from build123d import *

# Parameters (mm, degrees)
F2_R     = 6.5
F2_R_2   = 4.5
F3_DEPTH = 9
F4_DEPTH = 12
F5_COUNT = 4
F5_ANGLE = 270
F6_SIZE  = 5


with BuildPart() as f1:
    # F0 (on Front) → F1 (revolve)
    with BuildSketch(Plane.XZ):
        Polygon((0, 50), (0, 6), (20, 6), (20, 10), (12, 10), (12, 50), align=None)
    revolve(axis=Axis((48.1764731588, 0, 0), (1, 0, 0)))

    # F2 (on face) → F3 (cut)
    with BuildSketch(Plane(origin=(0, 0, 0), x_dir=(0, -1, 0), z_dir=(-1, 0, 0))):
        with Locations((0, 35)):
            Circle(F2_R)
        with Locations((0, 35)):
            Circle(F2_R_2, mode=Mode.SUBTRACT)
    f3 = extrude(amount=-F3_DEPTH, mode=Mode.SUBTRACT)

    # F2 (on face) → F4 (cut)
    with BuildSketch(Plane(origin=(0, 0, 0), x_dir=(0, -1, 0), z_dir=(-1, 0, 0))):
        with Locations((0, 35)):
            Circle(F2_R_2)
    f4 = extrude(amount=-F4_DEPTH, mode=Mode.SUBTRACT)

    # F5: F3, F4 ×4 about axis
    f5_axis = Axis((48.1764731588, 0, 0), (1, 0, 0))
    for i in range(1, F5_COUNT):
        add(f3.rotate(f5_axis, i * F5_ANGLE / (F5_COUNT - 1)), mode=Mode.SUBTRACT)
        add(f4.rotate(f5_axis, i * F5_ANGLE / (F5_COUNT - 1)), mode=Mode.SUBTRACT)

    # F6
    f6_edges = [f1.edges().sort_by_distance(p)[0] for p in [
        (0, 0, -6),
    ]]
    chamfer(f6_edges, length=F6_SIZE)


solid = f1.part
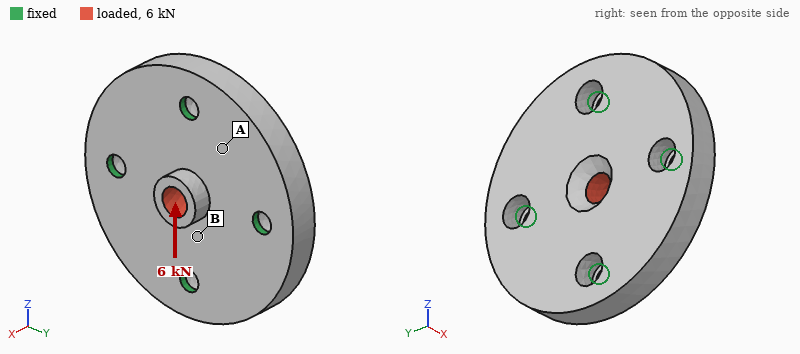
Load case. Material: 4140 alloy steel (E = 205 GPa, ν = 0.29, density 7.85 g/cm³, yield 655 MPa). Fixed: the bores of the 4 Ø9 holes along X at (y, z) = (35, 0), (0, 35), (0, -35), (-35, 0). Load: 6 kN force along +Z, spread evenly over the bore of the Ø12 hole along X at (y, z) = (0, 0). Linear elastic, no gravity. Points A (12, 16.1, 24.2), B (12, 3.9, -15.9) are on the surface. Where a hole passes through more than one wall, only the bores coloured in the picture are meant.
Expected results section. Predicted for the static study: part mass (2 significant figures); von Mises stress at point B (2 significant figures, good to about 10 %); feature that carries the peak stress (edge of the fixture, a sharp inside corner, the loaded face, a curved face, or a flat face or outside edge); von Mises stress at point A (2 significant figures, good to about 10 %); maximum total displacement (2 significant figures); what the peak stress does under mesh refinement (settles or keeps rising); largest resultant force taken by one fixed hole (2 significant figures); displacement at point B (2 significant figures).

690 g
19 MPa
edge of the fixture
5.5 MPa
5.9 µm
keeps rising
1.6 kN
1.7 µm
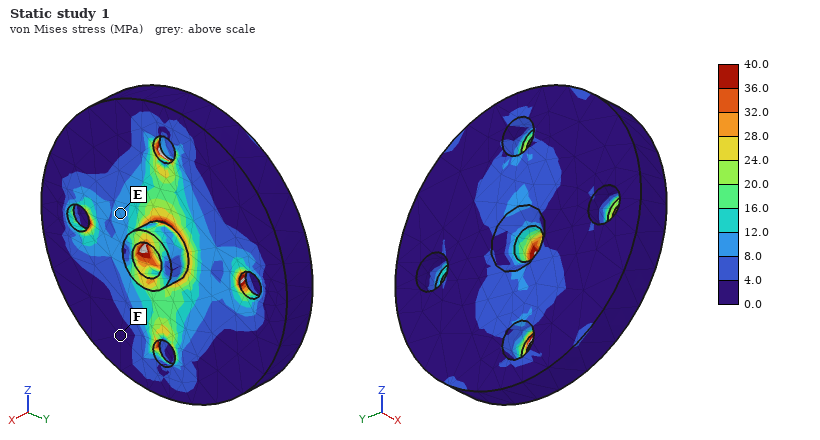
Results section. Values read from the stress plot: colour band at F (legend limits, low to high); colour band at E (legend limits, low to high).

0.0 to 4.0 MPa
8.0 to 12.0 MPa
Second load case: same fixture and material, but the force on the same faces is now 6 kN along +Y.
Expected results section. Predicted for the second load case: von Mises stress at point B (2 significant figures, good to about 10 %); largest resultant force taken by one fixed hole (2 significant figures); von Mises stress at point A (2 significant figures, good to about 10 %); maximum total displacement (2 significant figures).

10 MPa
1.6 kN
5.0 MPa
5.9 µm
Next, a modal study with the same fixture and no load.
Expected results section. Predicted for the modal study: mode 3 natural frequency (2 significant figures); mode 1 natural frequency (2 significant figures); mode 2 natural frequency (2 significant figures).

9400 Hz
8400 Hz
9400 Hz
